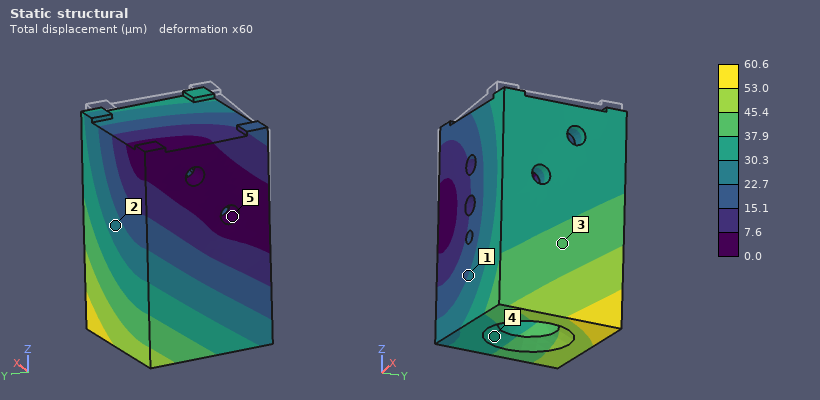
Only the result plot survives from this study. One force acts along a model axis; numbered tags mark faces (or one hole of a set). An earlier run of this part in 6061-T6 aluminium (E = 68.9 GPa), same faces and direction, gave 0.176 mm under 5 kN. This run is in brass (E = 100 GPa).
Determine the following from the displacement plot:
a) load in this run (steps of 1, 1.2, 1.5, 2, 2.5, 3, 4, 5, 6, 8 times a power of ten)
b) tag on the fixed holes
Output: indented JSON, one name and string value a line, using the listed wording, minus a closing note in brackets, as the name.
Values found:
{
  "load in this run": "2.5 kN",
  "tag on the fixed holes": "5"
}
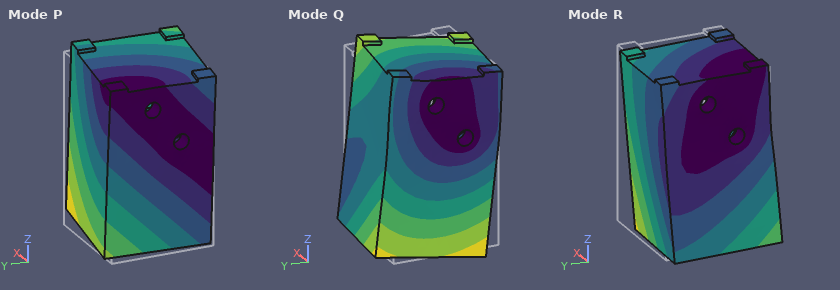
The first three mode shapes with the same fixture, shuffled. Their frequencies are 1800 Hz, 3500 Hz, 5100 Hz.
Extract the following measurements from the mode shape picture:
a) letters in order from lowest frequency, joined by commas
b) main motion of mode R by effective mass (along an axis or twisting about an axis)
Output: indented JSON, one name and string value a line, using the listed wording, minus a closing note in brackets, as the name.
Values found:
{
  "letters in order from lowest frequency, joined by commas": "P, R, Q",
  "main motion of mode R by effective mass": "along Y"
}
